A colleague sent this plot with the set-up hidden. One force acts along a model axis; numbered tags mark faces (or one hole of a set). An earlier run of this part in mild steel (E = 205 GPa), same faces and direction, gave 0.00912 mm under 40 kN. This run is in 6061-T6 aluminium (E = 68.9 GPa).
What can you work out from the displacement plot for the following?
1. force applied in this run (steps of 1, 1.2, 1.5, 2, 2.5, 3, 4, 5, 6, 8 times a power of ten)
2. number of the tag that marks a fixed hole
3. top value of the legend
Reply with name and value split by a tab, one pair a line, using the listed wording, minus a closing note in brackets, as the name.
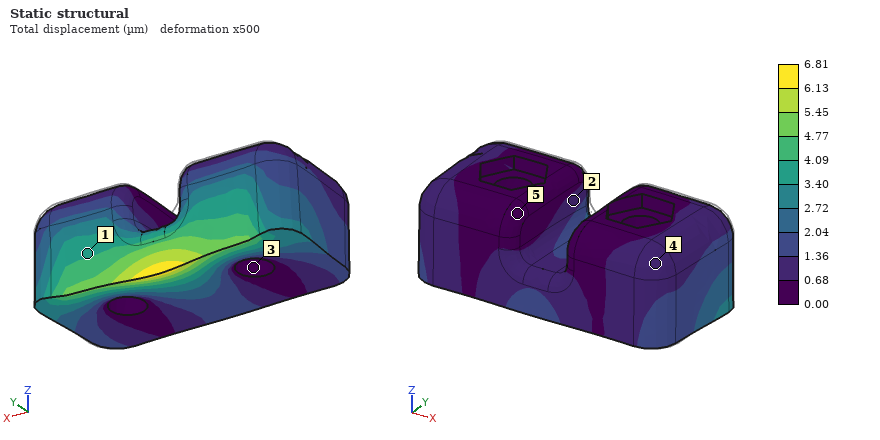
force applied in this run	10 kN
number of the tag that marks a fixed hole	3
top value of the legend	6.81 µm
